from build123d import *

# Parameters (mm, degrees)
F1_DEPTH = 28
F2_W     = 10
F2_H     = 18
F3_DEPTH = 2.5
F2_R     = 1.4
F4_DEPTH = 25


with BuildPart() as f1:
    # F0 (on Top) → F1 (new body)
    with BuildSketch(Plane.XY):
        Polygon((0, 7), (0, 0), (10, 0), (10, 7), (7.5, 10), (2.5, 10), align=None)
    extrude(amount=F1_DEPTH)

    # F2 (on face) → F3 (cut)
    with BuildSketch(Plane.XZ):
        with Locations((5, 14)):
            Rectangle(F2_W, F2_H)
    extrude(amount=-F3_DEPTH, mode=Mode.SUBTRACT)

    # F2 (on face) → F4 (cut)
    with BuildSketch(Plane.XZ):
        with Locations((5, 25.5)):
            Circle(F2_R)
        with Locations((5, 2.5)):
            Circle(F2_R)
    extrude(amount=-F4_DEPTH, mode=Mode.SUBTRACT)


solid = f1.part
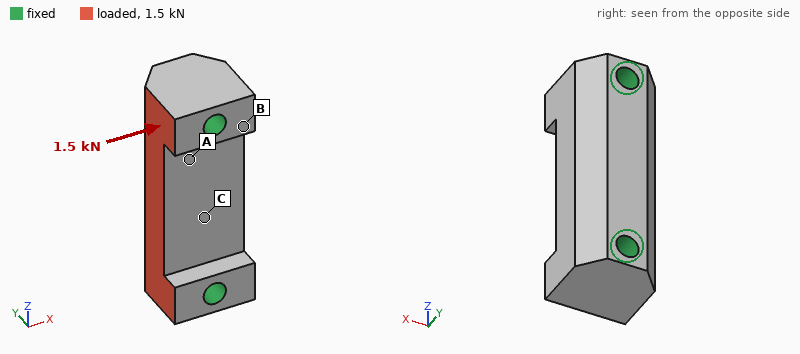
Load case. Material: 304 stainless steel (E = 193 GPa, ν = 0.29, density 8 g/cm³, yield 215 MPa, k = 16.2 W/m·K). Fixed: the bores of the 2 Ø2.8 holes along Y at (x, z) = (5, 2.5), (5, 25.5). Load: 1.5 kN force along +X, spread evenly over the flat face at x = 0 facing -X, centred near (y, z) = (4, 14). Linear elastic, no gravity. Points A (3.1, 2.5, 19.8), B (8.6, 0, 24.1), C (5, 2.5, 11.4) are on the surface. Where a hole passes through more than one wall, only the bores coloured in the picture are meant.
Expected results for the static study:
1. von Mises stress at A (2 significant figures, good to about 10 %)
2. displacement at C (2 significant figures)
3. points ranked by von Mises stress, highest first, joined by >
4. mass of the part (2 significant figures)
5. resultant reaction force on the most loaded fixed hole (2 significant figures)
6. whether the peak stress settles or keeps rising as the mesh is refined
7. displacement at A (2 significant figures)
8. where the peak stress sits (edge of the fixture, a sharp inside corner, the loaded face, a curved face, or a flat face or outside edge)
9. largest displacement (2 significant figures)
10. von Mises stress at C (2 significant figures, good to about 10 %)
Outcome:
16 MPa
1.3 µm
A > C > B
16 g
750 N
keeps rising
1.0 µm
edge of the fixture
1.7 µm
9.4 MPa
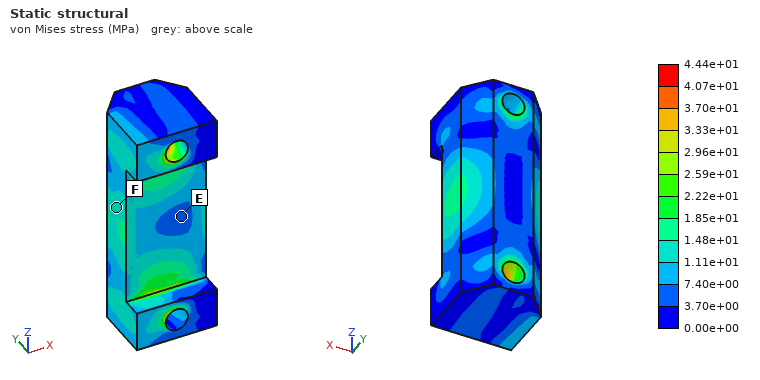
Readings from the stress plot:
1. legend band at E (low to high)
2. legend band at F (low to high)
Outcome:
3.70e+00 to 7.40e+00 MPa
1.11e+01 to 1.48e+01 MPa
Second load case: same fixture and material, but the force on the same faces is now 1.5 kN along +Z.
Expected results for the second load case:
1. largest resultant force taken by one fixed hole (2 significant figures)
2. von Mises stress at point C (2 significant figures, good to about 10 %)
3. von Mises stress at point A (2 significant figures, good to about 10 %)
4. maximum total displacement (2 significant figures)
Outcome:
790 N
8.2 MPa
15 MPa
1.4 µm
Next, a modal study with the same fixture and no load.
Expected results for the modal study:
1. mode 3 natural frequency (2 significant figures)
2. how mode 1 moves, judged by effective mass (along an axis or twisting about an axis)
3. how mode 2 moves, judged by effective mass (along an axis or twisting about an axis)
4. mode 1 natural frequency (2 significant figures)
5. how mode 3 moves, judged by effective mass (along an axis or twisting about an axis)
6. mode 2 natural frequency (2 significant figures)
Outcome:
65 kHz
along X
along Y
45 kHz
twisting about Z
50 kHz
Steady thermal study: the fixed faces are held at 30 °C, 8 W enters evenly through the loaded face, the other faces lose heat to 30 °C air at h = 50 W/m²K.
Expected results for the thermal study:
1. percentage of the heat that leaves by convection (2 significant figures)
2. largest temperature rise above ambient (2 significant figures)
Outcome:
4.1 %
24 K
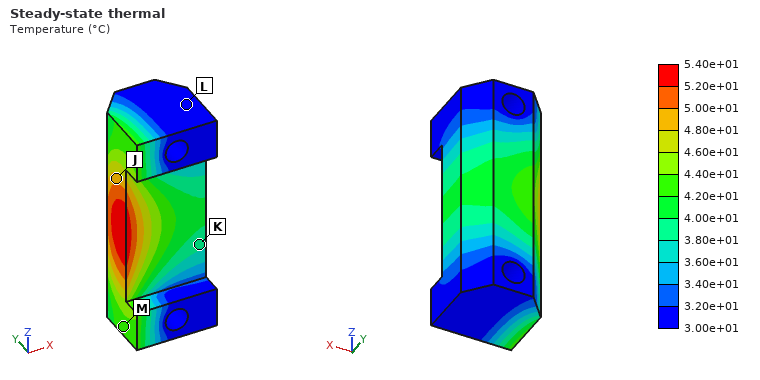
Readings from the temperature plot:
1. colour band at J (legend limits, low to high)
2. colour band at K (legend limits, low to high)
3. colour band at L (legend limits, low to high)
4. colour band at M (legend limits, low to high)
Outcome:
4.80e+01 to 5.00e+01 °C
3.80e+01 to 4.00e+01 °C
3.00e+01 to 3.20e+01 °C
4.20e+01 to 4.40e+01 °C
